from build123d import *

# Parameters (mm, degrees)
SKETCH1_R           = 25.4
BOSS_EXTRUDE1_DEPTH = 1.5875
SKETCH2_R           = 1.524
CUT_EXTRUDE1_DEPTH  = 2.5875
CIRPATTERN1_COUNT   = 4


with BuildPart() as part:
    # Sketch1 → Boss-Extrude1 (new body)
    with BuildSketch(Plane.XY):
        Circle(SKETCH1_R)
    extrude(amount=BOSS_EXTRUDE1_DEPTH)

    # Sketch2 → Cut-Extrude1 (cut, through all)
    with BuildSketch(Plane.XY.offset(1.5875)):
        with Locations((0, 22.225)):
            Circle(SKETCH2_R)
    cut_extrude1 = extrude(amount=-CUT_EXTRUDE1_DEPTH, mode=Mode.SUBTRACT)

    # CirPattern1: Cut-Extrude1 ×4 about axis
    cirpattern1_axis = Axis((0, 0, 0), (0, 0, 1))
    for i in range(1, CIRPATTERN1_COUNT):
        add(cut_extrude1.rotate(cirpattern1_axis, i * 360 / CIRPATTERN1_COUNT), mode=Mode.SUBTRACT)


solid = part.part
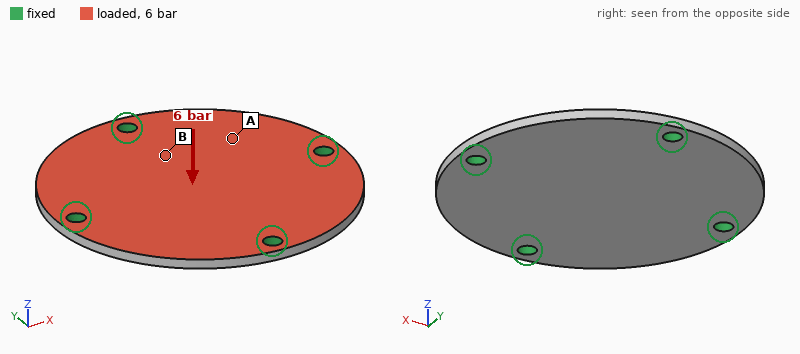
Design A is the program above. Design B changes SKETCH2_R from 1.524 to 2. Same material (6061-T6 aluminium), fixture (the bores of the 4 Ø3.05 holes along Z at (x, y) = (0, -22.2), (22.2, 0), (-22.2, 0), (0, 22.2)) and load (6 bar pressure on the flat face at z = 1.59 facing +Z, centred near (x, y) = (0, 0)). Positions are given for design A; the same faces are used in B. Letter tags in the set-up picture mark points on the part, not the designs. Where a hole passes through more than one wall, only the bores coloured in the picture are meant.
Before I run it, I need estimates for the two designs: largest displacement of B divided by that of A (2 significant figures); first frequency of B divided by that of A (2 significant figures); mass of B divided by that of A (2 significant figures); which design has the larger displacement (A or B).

0.88
1.1
0.99
A
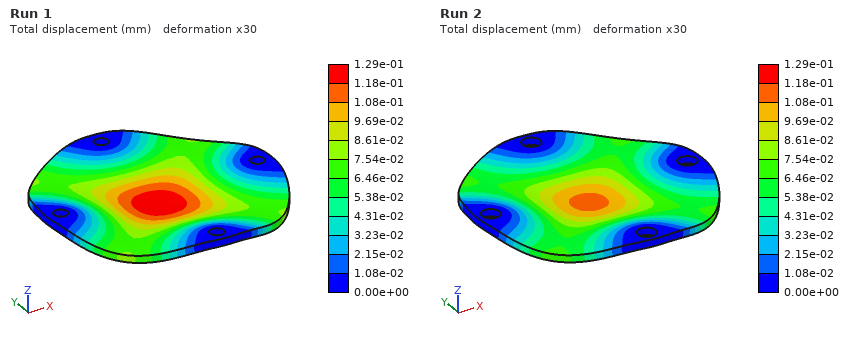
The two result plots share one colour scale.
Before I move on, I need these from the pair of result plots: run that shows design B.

Run 2
